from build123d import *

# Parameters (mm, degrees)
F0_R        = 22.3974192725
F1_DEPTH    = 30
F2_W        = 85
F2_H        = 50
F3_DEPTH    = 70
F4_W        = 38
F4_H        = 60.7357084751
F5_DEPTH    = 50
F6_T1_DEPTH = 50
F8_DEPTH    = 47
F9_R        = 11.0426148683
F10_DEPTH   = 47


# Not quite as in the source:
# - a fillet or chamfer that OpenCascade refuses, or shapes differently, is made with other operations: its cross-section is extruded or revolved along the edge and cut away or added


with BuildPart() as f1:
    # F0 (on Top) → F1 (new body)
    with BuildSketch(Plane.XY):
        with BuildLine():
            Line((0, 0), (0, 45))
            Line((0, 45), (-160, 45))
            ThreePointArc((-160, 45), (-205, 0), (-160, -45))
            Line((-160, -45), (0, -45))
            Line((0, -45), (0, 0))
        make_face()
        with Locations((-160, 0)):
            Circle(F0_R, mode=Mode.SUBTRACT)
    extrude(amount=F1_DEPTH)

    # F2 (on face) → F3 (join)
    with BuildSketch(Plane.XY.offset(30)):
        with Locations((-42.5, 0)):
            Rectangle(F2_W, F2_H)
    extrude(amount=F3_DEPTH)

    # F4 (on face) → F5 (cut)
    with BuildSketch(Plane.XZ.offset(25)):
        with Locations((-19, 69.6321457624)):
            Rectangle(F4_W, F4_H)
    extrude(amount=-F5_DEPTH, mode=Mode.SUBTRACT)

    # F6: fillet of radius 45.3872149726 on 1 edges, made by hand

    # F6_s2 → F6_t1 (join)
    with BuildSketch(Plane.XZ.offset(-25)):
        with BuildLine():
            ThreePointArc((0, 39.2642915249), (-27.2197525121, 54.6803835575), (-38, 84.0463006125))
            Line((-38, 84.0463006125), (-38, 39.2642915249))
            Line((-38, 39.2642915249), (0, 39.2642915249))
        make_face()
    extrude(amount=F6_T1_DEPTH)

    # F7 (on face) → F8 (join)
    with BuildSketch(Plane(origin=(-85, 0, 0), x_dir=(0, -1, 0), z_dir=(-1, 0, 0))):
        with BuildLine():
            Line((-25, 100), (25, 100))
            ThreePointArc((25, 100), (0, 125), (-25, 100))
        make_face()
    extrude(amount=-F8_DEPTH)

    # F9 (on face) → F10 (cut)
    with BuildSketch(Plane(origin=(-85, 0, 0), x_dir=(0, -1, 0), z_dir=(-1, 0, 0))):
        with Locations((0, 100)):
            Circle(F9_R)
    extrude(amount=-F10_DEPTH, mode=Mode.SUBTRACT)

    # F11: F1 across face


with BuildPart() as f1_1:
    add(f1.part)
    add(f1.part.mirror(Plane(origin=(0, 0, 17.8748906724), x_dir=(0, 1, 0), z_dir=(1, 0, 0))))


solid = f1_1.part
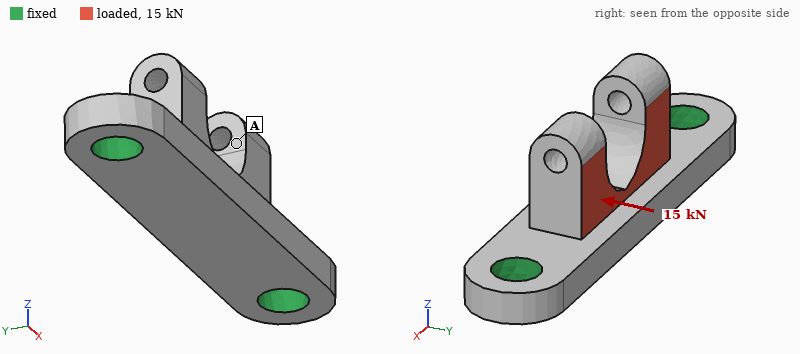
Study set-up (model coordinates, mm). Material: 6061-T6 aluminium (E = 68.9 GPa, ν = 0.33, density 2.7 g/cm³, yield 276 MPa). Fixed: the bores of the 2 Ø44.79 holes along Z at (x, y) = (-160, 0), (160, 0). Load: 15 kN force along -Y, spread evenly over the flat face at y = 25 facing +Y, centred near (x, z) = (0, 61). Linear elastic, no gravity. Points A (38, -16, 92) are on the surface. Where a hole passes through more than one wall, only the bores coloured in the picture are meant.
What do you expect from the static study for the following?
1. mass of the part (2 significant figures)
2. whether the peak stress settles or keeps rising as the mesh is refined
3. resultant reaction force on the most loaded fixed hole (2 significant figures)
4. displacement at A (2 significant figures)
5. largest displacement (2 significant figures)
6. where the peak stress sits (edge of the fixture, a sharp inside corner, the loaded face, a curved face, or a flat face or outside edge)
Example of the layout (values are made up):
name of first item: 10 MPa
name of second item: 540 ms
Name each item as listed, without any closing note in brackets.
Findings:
mass of the part: 3.8 kg
whether the peak stress settles or keeps rising as the mesh is refined: keeps rising
resultant reaction force on the most loaded fixed hole: 7.5 kN
displacement at A: 0.13 mm
largest displacement: 0.17 mm
where the peak stress sits: edge of the fixture
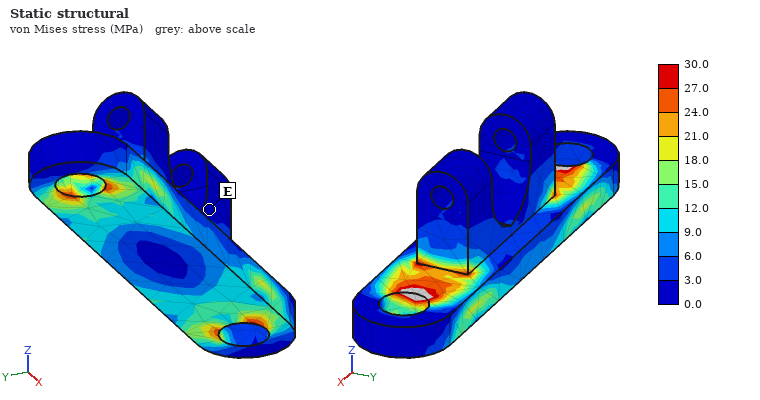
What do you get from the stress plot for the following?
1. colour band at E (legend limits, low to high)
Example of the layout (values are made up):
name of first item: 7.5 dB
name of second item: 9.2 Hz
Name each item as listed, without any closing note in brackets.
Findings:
colour band at E: 0.0 to 3.0 MPa
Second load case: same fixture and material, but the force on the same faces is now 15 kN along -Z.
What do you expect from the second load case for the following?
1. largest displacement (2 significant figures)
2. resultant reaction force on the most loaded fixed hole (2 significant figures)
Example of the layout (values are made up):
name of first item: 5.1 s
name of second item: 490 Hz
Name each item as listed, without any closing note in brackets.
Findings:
largest displacement: 0.11 mm
resultant reaction force on the most loaded fixed hole: 8.4 kN
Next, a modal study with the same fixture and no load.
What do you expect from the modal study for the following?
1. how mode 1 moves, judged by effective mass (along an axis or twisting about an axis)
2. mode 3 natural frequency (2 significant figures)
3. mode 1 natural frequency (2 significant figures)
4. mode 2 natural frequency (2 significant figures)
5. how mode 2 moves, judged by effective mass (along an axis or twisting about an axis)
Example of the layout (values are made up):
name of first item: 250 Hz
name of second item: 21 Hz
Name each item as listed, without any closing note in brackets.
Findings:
how mode 1 moves, judged by effective mass: along Y
mode 3 natural frequency: 2800 Hz
mode 1 natural frequency: 1400 Hz
mode 2 natural frequency: 1600 Hz
how mode 2 moves, judged by effective mass: along Z
